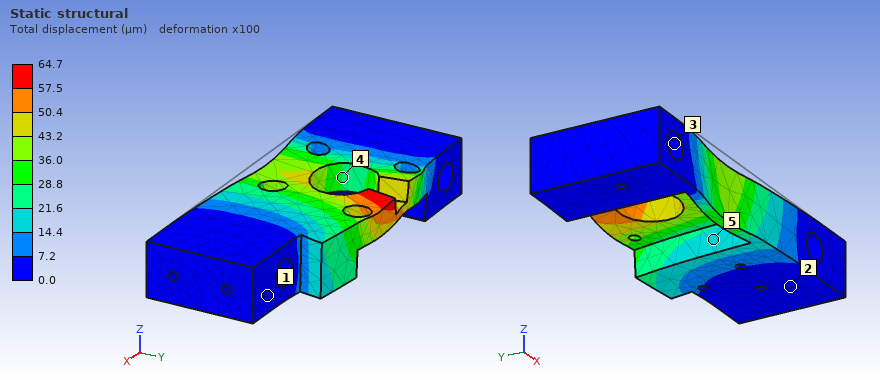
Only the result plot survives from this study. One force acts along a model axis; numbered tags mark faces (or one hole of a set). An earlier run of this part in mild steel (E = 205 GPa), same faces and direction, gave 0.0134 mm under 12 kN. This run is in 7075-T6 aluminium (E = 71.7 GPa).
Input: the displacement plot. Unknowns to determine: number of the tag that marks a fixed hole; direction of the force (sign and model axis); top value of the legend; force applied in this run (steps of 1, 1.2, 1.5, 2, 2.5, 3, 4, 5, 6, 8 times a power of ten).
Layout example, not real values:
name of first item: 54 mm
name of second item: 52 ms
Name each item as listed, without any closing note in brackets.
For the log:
number of the tag that marks a fixed hole: 3
direction of the force: +Y
top value of the legend: 64.7 µm
force applied in this run: 20 kN
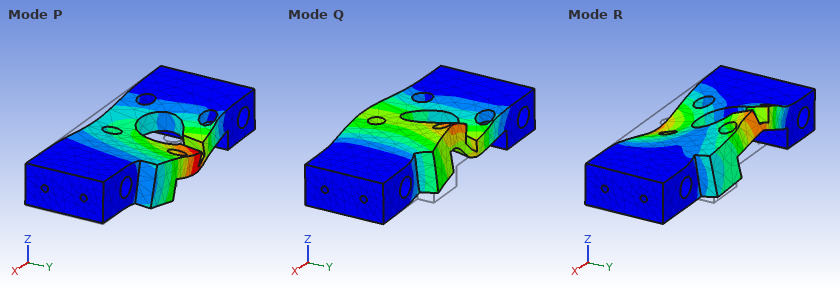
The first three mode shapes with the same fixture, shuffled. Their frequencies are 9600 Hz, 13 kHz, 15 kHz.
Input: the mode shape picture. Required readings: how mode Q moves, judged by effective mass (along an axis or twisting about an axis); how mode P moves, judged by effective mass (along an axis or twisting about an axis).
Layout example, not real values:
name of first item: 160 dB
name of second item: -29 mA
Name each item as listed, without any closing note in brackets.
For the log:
how mode Q moves, judged by effective mass: along Y
how mode P moves, judged by effective mass: along Z
